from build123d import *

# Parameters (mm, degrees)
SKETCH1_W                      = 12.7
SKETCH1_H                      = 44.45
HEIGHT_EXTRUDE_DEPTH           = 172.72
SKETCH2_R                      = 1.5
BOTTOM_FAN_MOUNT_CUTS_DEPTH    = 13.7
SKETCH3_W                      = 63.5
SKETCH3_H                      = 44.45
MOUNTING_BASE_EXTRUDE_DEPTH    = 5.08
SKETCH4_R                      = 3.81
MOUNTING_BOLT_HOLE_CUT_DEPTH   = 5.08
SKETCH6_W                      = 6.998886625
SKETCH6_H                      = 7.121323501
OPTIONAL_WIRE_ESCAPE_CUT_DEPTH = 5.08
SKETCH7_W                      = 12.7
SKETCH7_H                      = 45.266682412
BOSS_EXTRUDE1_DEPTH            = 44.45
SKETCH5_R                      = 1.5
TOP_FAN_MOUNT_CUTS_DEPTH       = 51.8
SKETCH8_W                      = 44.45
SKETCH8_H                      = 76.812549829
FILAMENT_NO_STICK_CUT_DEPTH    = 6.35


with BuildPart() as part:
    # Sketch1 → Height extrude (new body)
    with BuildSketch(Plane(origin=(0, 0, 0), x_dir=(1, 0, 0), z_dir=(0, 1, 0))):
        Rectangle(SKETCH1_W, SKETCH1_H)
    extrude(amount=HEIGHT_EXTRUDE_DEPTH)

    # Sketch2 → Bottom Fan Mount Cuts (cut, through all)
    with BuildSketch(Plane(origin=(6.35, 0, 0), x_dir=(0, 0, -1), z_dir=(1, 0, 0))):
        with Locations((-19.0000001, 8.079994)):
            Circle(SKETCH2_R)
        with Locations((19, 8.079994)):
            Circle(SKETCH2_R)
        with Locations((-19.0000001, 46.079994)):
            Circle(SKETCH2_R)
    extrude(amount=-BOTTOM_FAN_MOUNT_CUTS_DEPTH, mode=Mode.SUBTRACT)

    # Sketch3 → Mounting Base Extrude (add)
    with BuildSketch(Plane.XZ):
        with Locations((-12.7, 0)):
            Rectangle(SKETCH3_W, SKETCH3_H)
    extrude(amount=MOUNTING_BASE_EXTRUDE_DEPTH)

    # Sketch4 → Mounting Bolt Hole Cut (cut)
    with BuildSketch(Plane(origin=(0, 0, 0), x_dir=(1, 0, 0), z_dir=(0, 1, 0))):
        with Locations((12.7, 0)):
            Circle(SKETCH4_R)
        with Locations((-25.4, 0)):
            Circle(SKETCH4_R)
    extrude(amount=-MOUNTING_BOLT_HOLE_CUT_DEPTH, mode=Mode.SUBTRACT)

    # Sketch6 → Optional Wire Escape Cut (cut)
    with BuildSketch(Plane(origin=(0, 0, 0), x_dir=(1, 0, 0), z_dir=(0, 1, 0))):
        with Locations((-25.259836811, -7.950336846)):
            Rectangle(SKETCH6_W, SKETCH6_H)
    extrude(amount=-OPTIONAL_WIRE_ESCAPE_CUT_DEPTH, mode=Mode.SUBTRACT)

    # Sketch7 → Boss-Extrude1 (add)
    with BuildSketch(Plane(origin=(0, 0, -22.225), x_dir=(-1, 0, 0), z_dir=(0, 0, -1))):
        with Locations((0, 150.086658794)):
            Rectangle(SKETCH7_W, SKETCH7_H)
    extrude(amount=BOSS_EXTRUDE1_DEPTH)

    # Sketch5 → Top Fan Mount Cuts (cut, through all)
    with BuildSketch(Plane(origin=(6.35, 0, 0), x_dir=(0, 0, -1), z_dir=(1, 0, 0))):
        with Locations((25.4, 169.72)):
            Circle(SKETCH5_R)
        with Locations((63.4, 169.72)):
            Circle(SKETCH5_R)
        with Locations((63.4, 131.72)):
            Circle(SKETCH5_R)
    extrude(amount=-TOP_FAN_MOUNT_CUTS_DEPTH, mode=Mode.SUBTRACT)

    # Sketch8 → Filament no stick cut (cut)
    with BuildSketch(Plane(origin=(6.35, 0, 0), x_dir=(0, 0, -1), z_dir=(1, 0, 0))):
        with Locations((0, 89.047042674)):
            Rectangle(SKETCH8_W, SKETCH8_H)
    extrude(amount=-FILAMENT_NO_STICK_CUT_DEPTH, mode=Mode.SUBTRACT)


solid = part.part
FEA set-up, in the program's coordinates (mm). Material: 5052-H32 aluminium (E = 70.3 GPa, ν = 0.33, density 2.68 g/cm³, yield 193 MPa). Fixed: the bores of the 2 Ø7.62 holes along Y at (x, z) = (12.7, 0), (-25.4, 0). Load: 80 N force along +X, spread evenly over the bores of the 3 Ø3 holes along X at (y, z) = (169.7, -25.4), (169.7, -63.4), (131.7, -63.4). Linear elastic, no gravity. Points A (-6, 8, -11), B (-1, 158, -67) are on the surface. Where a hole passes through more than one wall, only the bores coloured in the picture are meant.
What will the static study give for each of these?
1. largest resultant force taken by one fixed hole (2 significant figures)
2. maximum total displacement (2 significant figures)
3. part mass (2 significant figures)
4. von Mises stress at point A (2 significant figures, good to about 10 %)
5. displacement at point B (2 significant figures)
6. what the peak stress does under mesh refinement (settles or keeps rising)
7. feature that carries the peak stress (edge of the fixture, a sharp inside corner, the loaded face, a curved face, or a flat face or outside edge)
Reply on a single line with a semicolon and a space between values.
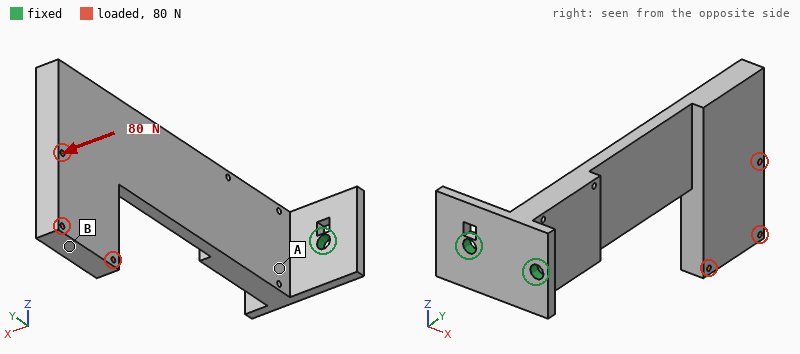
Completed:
430 N; 1.1 mm; 310 g; 11 MPa; 0.96 mm; keeps rising; edge of the fixture
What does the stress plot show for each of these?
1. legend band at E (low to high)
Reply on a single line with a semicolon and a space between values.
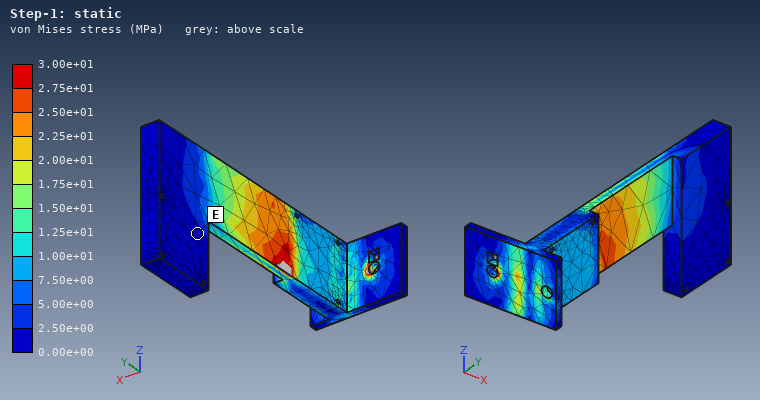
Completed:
0.00e+00 to 2.50e+00 MPa
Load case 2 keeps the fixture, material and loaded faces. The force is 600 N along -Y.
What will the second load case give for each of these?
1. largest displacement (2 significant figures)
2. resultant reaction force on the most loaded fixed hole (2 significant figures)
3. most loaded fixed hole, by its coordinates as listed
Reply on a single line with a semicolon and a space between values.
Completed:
0.67 mm; 420 N; (12.7, 0)
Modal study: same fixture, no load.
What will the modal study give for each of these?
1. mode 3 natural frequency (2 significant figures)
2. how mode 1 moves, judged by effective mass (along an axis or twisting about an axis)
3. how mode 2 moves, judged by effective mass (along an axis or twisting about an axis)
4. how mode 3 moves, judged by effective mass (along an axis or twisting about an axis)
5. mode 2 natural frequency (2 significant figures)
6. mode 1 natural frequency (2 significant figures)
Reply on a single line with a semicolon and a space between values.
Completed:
560 Hz; along X; along Z; twisting about Y; 250 Hz; 140 Hz
